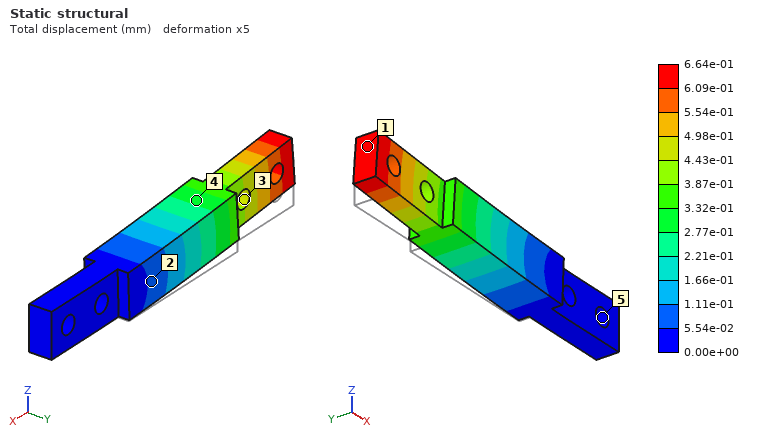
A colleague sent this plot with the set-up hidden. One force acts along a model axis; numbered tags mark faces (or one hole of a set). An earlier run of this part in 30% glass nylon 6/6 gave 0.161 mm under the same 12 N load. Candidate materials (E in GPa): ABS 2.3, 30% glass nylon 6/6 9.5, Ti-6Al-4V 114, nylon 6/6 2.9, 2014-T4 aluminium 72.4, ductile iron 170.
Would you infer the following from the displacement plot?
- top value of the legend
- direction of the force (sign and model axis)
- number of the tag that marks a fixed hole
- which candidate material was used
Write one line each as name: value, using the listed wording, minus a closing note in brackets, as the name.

top value of the legend: 6.64e-01 mm
direction of the force: +Z
number of the tag that marks a fixed hole: 5
which candidate material was used: ABS
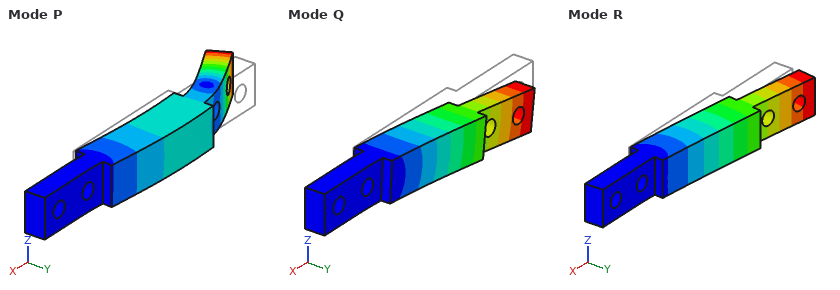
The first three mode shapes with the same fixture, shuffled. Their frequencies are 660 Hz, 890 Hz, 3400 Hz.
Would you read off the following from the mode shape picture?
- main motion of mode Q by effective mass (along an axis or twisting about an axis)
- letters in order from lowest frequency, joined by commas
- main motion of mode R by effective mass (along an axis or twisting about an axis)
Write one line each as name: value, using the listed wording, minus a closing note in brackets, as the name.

main motion of mode Q by effective mass: along Z
letters in order from lowest frequency, joined by commas: R, Q, P
main motion of mode R by effective mass: along Y
